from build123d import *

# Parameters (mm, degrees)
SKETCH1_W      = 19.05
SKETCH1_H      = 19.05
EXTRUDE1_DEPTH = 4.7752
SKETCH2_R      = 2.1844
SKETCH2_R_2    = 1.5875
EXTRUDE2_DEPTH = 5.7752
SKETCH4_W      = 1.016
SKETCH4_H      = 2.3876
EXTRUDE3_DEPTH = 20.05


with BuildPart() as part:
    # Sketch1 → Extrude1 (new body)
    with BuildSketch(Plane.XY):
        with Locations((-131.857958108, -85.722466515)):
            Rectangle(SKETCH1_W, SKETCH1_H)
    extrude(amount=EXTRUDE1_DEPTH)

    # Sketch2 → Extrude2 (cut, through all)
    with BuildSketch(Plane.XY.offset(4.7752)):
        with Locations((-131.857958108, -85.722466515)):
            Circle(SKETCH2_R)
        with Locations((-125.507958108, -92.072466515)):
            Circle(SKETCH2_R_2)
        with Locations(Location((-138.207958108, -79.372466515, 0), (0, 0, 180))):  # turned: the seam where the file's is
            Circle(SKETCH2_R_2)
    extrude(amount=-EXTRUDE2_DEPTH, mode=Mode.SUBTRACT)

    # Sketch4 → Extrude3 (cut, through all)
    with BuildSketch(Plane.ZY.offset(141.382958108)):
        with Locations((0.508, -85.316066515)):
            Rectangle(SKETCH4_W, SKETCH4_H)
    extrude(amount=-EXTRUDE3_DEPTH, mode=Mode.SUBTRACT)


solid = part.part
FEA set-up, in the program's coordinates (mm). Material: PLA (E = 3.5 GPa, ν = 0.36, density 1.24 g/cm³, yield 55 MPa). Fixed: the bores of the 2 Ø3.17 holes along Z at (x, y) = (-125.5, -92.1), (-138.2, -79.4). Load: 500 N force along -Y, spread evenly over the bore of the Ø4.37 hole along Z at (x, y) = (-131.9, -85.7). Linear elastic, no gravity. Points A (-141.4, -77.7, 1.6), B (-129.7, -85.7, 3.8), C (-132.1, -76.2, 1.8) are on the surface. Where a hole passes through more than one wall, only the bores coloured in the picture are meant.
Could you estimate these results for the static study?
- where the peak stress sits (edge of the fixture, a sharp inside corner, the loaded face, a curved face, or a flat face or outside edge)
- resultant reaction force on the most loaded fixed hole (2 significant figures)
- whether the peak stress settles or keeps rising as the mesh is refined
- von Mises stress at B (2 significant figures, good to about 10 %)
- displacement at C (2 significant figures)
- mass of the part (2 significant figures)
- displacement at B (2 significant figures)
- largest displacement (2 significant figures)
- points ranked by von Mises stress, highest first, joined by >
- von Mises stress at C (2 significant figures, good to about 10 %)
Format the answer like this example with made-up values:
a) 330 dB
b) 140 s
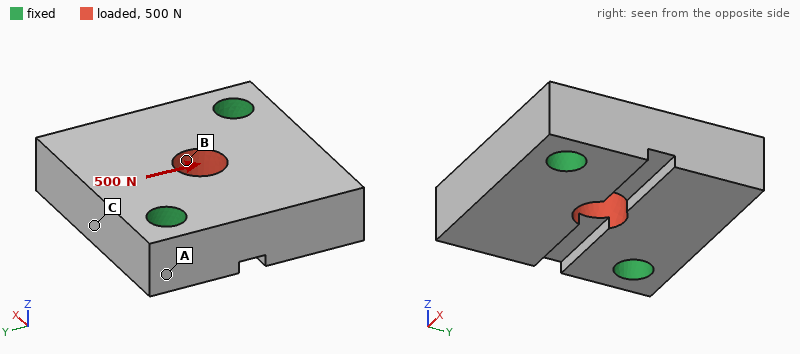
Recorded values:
a) edge of the fixture
b) 250 N
c) keeps rising
d) 15 MPa
e) 14 µm
f) 1.9 g
g) 23 µm
h) 26 µm
i) B > C > A
j) 6.0 MPa
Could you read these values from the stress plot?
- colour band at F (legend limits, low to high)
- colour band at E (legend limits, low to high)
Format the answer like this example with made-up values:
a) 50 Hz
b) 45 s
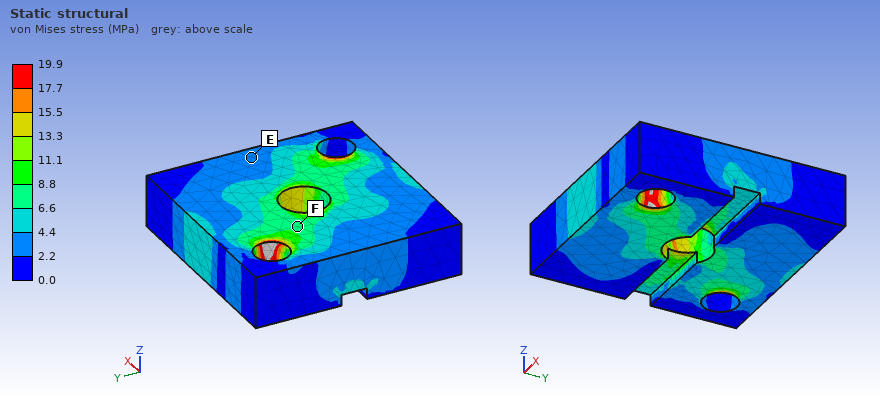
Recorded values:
a) 6.6 to 8.8 MPa
b) 2.2 to 4.4 MPa
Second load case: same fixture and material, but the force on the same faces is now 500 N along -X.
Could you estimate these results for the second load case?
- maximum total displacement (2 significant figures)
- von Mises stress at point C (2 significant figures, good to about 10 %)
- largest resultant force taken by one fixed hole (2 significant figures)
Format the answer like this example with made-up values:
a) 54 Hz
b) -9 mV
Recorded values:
a) 25 µm
b) 3.4 MPa
c) 250 N
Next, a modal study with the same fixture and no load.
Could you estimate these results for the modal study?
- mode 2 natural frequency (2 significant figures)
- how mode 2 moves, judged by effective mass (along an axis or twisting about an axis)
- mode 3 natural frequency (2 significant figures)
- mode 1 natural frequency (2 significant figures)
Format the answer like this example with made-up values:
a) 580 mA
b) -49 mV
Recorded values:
a) 9500 Hz
b) along Z
c) 22 kHz
d) 8000 Hz
